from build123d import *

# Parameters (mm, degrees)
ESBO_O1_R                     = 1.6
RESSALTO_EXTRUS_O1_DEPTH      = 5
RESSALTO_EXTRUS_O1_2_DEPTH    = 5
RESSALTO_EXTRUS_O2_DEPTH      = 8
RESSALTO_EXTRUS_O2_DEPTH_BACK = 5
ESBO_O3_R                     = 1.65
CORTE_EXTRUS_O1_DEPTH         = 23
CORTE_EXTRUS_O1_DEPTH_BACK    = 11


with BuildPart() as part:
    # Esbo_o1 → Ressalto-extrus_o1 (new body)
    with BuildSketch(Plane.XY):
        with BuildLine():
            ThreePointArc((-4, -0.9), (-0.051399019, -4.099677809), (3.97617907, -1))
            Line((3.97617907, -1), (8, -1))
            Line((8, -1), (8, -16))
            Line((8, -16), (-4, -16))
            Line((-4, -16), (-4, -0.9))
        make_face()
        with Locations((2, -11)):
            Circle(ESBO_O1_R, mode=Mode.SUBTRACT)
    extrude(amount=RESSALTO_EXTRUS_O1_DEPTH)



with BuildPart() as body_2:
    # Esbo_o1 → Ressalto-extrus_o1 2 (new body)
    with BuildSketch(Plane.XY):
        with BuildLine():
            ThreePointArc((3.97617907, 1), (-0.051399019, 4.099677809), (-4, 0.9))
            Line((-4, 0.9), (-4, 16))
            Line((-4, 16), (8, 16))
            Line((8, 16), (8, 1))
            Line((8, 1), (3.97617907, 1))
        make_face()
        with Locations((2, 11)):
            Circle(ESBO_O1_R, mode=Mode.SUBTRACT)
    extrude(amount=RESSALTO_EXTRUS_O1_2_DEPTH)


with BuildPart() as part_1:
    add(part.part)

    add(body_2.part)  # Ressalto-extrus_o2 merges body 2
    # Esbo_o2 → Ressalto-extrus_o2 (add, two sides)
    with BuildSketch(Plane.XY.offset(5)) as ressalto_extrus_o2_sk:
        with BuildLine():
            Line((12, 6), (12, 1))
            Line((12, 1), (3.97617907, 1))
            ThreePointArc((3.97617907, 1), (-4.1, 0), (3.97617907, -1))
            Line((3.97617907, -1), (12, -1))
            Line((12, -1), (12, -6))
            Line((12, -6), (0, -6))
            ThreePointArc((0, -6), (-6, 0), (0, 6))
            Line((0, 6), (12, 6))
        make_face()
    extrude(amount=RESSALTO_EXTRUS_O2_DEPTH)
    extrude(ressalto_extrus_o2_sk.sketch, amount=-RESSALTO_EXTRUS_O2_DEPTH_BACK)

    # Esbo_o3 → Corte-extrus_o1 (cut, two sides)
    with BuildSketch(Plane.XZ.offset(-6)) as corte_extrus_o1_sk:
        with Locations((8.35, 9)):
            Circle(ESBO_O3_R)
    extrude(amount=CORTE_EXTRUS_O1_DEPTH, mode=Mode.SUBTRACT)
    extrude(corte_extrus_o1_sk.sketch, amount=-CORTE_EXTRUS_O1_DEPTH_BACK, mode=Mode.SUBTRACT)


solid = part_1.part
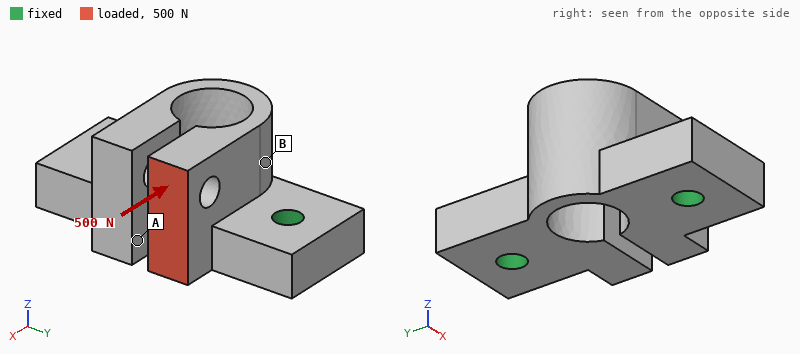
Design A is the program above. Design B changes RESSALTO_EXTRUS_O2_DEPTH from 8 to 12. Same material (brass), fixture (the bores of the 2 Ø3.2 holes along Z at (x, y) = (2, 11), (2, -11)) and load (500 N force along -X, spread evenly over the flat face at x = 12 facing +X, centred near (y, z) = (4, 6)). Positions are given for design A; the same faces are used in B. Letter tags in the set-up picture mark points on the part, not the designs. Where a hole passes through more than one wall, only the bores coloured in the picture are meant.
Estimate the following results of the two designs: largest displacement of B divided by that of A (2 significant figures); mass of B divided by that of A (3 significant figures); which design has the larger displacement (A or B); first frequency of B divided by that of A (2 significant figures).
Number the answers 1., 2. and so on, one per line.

1. 1.4
2. 1.19
3. B
4. 0.70
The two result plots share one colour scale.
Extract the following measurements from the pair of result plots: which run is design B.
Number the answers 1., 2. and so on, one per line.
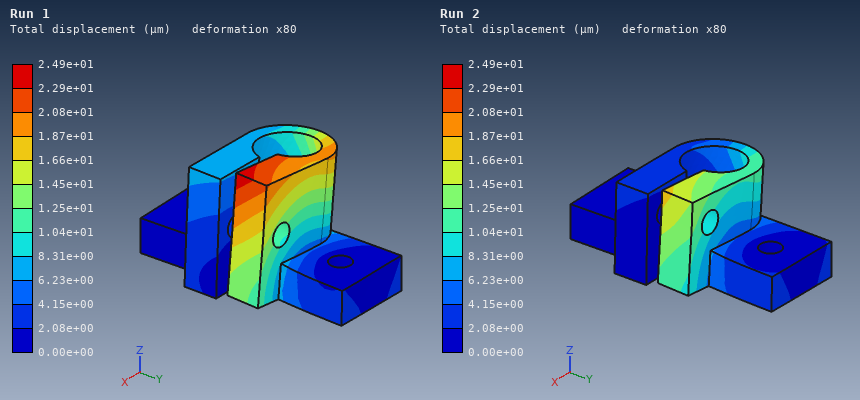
1. Run 1
